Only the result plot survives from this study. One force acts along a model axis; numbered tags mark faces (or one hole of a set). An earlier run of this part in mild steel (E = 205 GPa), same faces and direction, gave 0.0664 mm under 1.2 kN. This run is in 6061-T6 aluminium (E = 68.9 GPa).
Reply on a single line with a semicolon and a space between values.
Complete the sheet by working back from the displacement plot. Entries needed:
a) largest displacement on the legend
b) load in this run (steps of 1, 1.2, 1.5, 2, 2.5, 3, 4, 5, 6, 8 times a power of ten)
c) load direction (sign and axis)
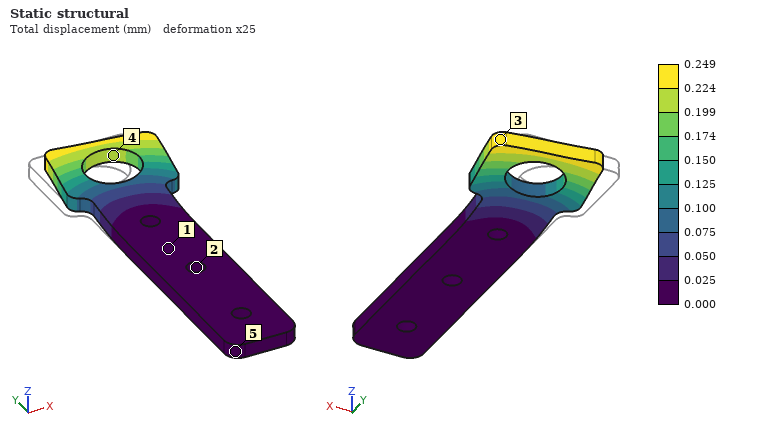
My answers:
0.249 mm; 1.5 kN; +X
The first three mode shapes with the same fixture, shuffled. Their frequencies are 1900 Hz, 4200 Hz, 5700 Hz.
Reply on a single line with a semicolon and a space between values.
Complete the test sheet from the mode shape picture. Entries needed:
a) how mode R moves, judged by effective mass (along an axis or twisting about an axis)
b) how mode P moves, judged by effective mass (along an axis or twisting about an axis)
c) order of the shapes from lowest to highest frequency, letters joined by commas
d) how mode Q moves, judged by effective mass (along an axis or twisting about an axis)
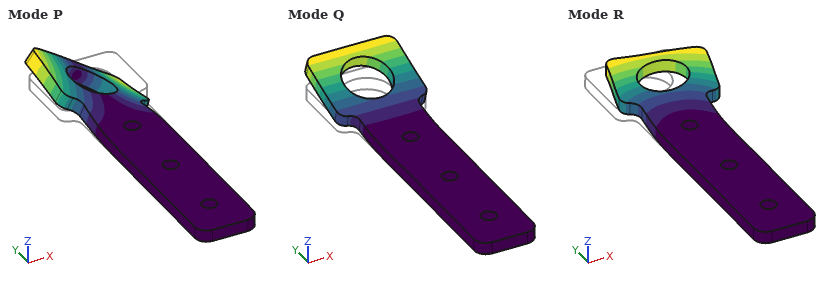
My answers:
along X; twisting about Y; Q, P, R; along Z
